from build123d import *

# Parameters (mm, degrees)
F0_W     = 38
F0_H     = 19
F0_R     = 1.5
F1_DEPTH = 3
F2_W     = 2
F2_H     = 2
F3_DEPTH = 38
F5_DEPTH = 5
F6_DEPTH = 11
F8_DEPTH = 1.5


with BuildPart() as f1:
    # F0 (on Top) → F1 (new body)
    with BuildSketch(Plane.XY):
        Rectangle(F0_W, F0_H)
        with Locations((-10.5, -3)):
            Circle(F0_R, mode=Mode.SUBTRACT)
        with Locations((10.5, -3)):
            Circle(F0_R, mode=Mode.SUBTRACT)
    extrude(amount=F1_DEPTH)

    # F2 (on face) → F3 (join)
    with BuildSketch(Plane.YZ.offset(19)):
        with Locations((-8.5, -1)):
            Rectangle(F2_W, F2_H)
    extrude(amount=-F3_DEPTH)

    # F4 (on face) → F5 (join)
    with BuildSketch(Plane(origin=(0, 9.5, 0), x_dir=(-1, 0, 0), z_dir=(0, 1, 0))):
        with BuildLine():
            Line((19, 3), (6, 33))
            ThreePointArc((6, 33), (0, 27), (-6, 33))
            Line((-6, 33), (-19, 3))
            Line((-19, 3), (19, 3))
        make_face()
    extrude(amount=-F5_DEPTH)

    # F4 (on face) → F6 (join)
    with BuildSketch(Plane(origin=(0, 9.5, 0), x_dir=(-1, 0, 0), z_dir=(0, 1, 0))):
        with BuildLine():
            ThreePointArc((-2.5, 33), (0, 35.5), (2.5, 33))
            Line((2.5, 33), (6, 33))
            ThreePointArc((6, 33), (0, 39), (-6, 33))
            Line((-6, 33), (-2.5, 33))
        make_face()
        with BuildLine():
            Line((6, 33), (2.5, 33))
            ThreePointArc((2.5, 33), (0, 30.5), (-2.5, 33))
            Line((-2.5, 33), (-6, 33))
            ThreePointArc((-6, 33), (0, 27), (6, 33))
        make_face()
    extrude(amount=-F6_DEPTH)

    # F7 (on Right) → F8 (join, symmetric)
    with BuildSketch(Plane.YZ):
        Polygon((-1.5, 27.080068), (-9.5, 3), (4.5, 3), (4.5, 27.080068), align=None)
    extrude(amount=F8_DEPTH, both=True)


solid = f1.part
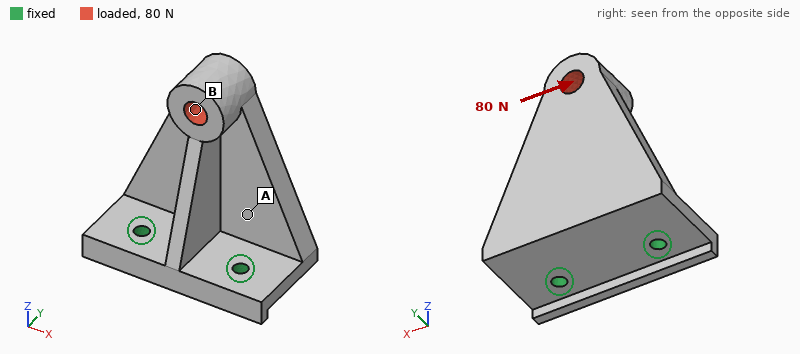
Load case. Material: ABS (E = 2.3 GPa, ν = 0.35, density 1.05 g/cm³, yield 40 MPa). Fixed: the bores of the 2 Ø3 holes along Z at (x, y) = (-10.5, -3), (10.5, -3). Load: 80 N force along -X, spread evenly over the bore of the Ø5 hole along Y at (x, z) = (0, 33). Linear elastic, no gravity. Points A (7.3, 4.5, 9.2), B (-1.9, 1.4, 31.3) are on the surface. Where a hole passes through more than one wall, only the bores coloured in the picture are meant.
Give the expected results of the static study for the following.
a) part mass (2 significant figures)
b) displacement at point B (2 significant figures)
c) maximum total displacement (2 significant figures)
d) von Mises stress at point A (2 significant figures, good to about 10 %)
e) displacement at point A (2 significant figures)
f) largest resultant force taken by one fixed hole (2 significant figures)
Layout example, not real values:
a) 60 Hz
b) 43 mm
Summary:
a) 7.9 g
b) 0.49 mm
c) 0.64 mm
d) 5.1 MPa
e) 0.15 mm
f) 120 N
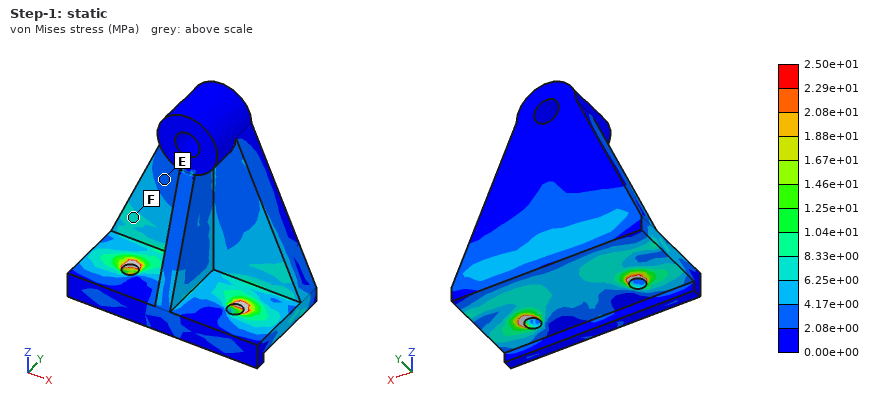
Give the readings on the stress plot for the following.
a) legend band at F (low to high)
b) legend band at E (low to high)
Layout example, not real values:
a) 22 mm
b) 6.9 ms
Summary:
a) 6.25e+00 to 8.33e+00 MPa
b) 2.08e+00 to 4.17e+00 MPa
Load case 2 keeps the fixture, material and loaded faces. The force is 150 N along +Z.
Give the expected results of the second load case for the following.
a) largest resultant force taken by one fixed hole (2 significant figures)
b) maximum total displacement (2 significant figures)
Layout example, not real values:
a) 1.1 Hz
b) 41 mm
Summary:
a) 75 N
b) 0.56 mm
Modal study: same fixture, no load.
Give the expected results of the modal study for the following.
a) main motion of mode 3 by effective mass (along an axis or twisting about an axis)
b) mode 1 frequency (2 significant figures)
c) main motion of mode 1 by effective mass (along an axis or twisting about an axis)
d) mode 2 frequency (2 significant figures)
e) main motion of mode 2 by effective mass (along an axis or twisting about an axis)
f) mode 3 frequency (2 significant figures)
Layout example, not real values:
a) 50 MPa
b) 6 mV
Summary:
a) along Z
b) 730 Hz
c) along Y
d) 1400 Hz
e) along X
f) 3200 Hz
